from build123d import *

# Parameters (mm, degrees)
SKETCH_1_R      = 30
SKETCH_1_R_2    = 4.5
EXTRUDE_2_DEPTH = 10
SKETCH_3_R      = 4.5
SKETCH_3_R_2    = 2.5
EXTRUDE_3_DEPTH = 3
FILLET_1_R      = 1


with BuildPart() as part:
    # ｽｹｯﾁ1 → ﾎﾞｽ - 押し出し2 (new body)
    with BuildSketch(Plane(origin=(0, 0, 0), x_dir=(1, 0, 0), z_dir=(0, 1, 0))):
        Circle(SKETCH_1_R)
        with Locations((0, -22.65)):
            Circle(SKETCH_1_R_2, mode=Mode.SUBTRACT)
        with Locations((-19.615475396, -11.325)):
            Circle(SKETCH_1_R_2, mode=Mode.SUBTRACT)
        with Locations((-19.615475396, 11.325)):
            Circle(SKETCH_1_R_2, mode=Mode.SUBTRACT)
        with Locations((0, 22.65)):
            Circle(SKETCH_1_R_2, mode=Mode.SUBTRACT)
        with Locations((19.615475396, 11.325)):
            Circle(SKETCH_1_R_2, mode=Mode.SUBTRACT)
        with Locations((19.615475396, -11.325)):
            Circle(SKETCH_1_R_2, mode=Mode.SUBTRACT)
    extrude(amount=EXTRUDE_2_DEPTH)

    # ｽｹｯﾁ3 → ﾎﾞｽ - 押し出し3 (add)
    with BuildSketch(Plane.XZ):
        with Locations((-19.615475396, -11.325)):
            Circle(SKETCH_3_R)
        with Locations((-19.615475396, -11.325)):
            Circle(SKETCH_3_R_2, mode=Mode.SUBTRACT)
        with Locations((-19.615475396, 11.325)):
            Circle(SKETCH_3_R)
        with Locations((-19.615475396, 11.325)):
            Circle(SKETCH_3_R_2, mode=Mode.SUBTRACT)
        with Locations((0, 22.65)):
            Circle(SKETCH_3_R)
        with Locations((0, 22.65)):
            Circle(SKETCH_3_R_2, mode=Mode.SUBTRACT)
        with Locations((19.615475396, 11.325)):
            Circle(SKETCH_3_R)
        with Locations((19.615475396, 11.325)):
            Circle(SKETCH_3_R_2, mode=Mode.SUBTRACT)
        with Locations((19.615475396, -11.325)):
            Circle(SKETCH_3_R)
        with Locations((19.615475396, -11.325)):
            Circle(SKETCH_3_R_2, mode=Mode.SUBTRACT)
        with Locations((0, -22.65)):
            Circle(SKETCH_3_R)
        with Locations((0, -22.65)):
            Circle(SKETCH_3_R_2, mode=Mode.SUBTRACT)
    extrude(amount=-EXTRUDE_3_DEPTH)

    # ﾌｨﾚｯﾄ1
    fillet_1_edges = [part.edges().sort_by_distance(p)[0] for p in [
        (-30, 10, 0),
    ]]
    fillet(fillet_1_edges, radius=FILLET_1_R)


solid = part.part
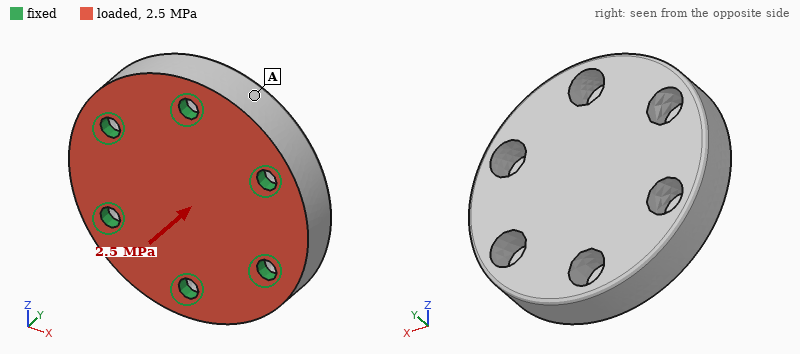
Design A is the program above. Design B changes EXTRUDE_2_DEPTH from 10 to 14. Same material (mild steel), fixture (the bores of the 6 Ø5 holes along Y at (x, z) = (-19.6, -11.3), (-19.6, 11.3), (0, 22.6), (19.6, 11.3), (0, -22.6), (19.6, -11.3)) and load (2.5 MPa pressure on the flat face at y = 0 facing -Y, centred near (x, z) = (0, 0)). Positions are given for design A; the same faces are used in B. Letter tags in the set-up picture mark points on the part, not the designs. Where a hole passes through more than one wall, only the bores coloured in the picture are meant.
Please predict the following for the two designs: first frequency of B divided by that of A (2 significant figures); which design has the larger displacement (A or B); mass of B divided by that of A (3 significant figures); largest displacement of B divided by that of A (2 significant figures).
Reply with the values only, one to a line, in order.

0.94
A
1.39
0.74
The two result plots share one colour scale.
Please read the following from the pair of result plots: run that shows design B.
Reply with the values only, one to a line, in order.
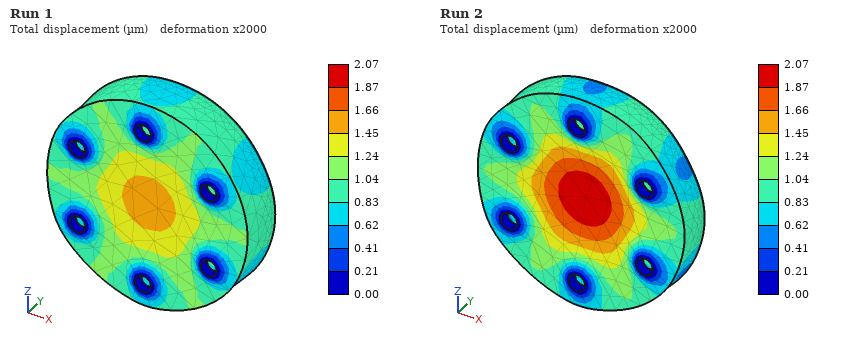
Run 1
